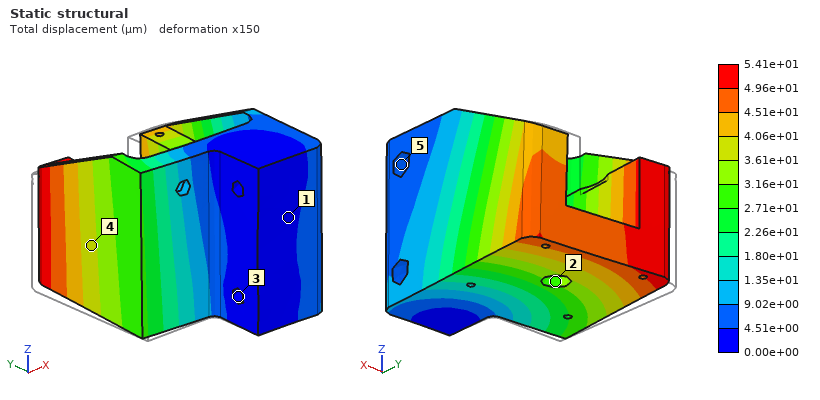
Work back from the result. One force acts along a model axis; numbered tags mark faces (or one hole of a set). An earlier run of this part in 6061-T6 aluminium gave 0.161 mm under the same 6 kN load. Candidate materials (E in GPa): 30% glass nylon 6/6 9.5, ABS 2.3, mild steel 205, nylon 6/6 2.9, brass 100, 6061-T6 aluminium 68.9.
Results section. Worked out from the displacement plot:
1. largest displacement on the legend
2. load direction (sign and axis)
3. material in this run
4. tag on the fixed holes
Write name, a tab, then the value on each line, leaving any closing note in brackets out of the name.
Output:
largest displacement on the legend	5.41e+01 µm
load direction	+X
material in this run	mild steel
tag on the fixed holes	3
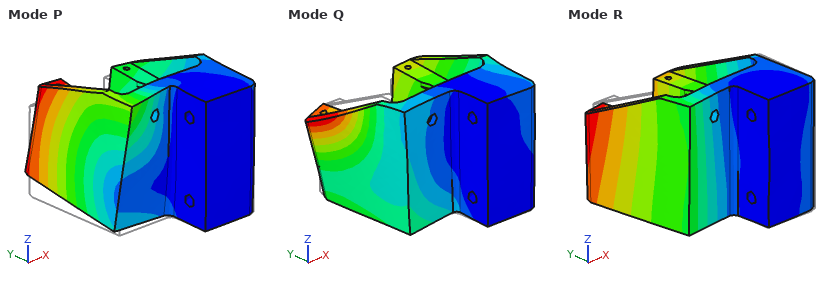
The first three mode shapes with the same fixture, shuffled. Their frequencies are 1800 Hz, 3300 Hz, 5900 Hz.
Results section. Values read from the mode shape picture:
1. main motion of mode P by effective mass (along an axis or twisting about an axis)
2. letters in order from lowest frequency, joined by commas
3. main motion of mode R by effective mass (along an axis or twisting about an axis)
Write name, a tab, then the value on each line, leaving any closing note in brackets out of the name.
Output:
main motion of mode P by effective mass	along Z
letters in order from lowest frequency, joined by commas	R, P, Q
main motion of mode R by effective mass	along X
